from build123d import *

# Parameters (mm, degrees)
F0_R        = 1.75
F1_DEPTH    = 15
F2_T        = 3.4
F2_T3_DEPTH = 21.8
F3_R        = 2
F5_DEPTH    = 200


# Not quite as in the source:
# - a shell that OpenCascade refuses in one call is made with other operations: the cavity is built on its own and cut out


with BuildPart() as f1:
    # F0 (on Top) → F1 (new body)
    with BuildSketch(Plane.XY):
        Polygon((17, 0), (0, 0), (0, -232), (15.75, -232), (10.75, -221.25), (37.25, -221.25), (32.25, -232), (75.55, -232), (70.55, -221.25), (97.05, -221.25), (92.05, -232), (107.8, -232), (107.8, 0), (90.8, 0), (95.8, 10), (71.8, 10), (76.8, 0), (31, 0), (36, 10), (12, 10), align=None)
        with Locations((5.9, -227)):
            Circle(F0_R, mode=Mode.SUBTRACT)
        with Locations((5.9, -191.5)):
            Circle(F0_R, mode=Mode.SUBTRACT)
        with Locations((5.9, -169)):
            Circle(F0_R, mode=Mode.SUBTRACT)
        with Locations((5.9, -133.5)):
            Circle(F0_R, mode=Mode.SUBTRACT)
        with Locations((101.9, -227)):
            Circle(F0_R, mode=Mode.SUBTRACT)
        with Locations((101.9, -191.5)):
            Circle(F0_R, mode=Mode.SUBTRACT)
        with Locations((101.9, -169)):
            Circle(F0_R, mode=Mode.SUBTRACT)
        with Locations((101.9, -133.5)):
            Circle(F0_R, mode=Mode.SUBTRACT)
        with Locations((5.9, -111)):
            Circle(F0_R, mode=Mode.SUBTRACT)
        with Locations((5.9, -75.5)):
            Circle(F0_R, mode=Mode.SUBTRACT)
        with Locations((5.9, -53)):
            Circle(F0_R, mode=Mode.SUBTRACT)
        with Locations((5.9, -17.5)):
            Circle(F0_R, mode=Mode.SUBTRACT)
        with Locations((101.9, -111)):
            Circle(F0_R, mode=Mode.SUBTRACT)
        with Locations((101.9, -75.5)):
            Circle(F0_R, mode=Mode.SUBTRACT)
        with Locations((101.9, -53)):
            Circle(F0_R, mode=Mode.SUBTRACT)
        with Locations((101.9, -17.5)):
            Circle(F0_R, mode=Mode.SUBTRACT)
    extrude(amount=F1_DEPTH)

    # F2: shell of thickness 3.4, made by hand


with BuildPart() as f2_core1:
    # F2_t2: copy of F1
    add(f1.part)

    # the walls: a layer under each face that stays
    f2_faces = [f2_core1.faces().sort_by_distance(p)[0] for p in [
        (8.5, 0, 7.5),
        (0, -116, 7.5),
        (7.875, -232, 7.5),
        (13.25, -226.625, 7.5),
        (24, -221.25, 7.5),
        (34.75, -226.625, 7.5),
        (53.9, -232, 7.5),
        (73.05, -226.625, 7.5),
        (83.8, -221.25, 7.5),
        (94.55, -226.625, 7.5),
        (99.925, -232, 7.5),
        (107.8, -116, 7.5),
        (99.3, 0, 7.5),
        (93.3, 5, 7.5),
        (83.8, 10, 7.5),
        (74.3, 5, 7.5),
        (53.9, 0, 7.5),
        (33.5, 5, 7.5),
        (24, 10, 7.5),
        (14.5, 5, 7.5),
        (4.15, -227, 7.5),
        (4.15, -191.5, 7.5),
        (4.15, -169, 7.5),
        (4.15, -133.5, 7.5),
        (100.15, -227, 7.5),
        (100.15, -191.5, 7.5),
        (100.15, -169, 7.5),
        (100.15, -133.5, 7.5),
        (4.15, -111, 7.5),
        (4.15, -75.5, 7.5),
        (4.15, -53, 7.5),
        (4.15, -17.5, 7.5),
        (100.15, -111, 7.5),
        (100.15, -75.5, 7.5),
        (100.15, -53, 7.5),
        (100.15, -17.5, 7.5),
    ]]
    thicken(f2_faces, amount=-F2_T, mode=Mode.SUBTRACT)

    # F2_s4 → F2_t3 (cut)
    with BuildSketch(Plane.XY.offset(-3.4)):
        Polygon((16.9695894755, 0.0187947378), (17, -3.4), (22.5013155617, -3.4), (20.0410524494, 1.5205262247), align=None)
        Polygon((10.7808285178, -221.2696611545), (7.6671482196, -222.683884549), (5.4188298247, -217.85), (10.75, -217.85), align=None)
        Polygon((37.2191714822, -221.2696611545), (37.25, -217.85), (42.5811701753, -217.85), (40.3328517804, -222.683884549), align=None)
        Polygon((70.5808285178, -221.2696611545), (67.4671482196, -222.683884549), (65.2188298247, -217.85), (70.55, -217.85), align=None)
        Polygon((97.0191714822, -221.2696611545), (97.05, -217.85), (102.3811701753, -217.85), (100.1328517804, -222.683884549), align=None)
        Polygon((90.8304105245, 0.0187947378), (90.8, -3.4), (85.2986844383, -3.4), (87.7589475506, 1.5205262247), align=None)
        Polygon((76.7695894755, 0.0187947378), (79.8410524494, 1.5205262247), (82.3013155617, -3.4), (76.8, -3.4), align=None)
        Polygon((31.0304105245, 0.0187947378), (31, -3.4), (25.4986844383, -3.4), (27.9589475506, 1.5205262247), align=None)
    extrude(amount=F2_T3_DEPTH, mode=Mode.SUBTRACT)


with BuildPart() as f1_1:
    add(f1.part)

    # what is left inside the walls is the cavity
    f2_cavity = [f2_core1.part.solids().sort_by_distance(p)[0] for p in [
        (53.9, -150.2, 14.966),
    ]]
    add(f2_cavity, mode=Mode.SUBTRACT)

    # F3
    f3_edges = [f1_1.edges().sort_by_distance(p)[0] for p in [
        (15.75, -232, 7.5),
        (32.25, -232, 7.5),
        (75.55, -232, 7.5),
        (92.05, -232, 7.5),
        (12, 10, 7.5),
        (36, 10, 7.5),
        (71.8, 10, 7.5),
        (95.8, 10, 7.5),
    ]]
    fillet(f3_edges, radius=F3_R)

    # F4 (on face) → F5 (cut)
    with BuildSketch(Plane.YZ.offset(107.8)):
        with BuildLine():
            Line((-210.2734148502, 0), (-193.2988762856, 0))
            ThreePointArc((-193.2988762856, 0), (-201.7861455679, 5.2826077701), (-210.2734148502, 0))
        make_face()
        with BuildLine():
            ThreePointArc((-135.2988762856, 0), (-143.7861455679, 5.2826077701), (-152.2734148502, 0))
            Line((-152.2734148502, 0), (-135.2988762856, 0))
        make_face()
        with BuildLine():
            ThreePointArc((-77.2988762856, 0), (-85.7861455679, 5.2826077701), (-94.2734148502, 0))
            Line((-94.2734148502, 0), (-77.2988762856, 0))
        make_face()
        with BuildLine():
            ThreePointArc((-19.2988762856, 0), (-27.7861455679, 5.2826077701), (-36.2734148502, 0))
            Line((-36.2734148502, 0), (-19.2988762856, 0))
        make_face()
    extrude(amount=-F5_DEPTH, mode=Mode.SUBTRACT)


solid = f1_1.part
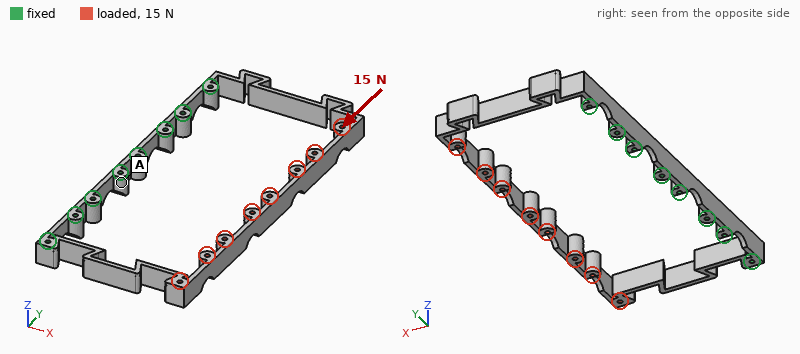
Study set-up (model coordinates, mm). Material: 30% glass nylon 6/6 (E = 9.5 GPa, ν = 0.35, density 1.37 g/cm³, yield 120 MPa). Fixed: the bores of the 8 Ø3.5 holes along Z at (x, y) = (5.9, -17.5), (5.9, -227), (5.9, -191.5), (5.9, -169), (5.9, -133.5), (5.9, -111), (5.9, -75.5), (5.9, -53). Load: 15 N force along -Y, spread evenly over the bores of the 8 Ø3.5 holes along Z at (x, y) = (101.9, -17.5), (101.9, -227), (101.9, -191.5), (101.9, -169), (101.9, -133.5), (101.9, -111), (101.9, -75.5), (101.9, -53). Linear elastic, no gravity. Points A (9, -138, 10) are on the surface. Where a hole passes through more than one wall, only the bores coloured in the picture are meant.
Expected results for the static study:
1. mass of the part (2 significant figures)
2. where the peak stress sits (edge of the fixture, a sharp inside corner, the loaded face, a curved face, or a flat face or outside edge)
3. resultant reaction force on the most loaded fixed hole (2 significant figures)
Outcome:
70 g
a curved face
15 N
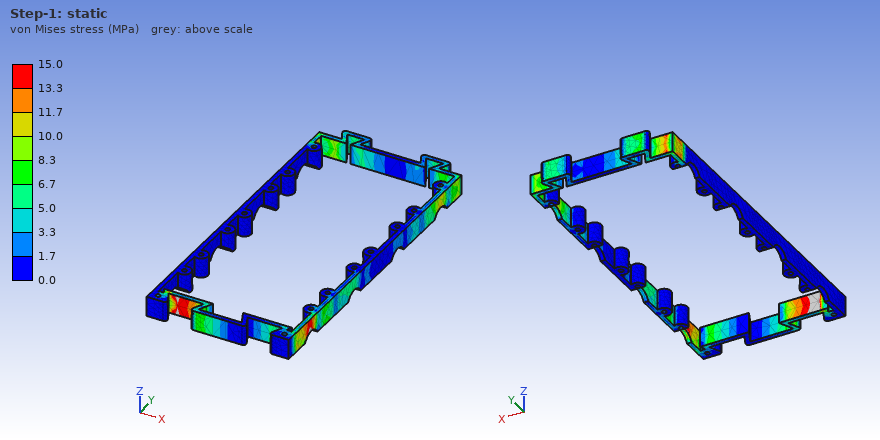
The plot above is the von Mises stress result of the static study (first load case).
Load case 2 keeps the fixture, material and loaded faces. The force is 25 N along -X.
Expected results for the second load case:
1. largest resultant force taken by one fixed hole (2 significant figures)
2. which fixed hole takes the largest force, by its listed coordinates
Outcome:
17 N
(5.9, -17.5)
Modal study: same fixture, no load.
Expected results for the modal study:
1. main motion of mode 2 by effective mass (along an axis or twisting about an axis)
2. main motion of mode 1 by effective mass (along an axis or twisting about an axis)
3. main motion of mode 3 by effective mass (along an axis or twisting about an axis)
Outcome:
along Z
along Y
along X
